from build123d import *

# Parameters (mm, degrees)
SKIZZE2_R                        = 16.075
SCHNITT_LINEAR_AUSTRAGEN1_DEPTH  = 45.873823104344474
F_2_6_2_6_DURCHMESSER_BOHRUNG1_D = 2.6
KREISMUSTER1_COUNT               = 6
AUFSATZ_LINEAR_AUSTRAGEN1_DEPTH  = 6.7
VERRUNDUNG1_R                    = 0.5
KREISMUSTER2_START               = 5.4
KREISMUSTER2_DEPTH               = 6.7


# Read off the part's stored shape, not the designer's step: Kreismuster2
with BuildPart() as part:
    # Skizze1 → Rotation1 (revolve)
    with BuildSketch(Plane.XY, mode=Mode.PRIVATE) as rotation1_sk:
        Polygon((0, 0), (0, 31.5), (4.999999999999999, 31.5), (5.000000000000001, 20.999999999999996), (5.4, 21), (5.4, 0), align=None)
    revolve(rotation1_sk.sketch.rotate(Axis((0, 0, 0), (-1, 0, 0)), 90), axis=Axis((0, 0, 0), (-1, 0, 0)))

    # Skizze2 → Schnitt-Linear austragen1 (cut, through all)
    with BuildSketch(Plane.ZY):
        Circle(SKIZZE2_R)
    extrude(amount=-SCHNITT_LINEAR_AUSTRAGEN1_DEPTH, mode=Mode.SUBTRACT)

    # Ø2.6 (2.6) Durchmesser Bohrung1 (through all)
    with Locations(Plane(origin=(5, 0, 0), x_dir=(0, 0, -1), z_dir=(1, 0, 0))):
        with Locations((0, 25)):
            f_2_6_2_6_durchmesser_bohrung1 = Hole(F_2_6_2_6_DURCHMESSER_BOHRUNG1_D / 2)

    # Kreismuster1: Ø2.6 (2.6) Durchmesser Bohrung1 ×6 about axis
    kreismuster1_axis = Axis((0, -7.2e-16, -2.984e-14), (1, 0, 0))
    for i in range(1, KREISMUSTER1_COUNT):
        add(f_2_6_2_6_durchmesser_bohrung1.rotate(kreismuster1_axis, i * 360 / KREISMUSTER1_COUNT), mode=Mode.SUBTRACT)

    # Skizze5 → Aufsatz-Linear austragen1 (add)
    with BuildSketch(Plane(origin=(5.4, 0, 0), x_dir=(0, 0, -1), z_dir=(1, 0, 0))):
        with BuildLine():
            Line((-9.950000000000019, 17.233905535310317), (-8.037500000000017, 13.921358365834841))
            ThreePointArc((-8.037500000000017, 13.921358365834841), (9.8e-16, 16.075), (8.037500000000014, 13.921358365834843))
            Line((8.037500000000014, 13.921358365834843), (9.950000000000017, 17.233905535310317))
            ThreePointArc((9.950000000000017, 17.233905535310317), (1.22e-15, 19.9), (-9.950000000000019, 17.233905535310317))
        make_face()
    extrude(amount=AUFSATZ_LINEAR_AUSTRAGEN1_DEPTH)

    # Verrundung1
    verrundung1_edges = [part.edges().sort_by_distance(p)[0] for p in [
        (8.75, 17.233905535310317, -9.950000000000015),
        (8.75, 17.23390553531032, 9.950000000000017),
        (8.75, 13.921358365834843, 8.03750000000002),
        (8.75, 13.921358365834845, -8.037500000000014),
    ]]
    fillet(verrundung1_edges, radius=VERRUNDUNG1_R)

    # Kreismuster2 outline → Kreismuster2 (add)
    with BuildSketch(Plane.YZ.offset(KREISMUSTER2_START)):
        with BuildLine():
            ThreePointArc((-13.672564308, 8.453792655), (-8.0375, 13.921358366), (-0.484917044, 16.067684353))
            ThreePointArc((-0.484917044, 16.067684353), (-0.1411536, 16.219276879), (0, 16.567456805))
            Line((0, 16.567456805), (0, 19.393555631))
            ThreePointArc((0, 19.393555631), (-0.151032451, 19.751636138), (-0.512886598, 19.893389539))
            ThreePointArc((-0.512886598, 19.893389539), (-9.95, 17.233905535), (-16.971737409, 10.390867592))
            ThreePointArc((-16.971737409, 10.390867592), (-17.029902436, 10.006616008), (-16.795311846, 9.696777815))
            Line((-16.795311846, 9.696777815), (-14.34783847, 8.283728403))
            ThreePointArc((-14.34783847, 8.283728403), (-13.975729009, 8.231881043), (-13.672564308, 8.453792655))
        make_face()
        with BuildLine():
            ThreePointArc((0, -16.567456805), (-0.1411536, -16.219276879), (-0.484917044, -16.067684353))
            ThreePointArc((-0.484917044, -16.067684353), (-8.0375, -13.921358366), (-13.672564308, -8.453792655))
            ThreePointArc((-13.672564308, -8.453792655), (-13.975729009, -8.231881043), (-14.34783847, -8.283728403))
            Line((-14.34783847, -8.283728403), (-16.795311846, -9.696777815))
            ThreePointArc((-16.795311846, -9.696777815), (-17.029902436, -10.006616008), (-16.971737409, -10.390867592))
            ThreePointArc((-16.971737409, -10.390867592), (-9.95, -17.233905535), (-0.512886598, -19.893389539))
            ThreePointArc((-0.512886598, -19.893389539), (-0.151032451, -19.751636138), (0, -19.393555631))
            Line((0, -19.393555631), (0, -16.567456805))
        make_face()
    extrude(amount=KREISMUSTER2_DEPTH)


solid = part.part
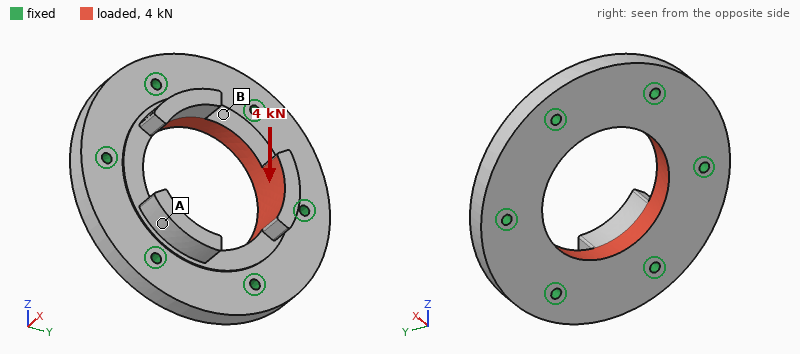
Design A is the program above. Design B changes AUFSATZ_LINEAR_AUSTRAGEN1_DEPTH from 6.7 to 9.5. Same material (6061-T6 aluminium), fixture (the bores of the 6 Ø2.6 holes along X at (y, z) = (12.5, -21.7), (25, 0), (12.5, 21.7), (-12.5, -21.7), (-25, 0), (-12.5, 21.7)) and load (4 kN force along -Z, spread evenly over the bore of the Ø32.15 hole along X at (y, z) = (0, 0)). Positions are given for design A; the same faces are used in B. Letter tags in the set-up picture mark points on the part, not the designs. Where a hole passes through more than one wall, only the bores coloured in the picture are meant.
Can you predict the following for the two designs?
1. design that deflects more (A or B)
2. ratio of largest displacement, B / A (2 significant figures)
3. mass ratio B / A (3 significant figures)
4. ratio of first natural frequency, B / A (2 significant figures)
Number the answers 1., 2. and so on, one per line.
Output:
1. B
2. 1.7
3. 1.02
4. 0.83
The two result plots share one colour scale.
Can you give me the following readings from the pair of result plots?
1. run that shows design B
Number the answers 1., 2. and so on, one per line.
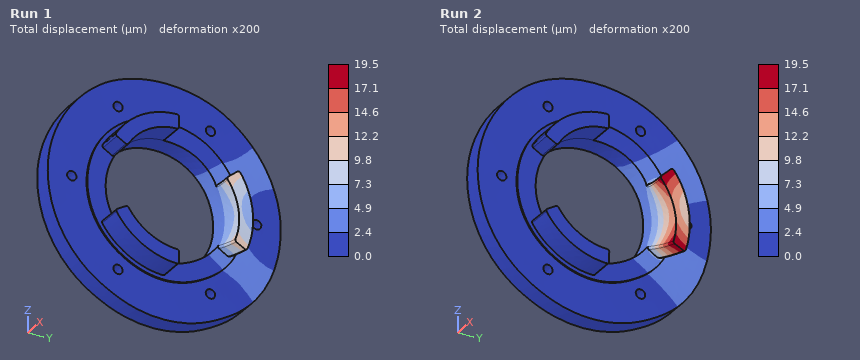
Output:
1. Run 2
